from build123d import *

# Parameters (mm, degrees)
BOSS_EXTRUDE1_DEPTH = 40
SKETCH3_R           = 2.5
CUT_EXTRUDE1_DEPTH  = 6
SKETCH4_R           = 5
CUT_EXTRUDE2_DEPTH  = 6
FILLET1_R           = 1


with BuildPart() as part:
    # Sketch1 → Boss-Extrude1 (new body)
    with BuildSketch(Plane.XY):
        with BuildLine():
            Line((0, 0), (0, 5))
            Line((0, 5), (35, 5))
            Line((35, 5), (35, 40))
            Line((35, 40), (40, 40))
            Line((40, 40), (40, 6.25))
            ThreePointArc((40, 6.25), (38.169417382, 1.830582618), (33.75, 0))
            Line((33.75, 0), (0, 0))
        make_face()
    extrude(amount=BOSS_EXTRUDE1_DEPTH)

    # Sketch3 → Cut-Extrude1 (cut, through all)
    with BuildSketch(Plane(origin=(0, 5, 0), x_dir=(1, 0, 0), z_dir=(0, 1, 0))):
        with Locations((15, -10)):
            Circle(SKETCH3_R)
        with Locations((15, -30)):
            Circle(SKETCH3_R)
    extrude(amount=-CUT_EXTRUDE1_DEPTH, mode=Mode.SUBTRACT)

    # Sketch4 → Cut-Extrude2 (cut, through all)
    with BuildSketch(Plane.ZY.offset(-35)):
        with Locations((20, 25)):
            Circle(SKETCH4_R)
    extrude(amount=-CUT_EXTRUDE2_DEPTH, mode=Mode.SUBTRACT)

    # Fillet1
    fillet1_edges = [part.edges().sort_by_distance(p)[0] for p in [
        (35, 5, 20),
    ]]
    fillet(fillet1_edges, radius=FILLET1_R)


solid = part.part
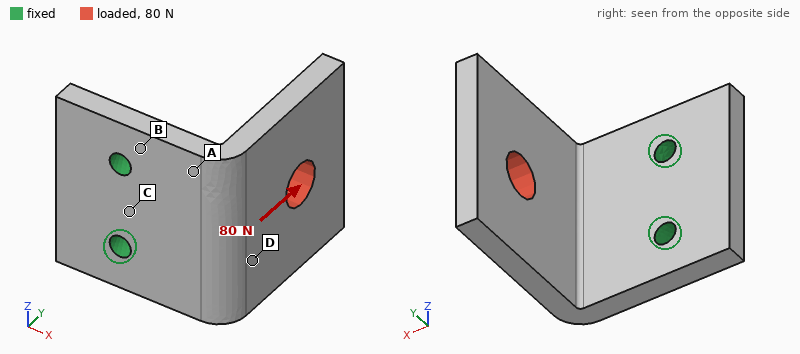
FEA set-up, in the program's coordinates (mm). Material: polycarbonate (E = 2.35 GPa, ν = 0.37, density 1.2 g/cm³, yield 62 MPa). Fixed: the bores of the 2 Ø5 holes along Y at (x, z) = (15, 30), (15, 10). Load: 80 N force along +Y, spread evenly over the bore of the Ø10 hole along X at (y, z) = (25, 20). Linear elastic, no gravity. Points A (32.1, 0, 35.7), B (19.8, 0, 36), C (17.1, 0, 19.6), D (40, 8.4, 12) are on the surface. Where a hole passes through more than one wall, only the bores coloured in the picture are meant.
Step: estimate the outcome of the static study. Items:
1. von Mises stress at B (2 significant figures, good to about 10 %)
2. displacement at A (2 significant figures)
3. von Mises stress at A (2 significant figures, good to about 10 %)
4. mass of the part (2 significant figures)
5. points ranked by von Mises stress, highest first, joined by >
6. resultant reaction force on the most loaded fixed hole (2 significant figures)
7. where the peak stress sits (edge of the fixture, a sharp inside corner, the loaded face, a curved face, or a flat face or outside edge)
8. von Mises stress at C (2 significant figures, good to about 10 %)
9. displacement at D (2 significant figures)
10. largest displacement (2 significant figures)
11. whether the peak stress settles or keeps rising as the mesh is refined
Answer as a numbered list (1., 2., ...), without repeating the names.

1. 6.5 MPa
2. 0.19 mm
3. 2.4 MPa
4. 17 g
5. B > C > A > D
6. 40 N
7. edge of the fixture
8. 4.9 MPa
9. 0.35 mm
10. 0.78 mm
11. keeps rising
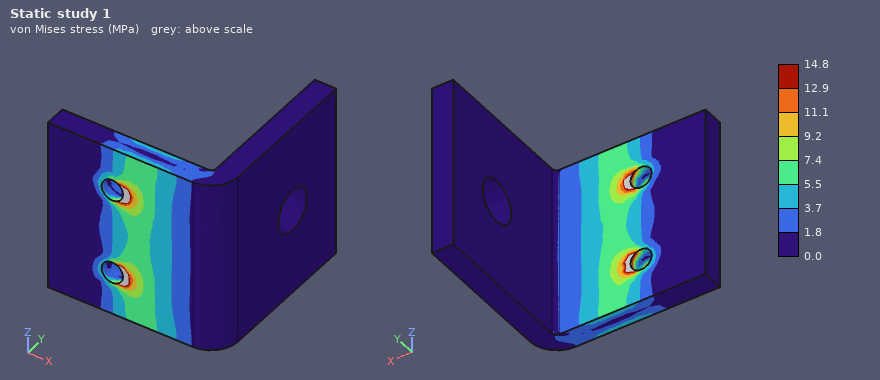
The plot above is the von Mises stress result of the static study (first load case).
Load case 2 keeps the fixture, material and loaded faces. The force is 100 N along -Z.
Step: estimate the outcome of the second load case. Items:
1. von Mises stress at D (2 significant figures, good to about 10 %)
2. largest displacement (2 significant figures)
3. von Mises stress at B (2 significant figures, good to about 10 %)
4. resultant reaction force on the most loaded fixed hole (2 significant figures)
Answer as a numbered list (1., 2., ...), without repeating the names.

1. 2.9 MPa
2. 0.80 mm
3. 8.0 MPa
4. 140 N
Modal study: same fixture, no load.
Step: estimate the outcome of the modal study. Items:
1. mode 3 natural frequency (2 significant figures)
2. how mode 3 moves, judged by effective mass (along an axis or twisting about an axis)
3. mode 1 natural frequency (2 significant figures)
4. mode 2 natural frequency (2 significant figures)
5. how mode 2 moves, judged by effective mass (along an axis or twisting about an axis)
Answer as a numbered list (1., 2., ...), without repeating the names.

1. 1300 Hz
2. along Y
3. 440 Hz
4. 760 Hz
5. along Z
